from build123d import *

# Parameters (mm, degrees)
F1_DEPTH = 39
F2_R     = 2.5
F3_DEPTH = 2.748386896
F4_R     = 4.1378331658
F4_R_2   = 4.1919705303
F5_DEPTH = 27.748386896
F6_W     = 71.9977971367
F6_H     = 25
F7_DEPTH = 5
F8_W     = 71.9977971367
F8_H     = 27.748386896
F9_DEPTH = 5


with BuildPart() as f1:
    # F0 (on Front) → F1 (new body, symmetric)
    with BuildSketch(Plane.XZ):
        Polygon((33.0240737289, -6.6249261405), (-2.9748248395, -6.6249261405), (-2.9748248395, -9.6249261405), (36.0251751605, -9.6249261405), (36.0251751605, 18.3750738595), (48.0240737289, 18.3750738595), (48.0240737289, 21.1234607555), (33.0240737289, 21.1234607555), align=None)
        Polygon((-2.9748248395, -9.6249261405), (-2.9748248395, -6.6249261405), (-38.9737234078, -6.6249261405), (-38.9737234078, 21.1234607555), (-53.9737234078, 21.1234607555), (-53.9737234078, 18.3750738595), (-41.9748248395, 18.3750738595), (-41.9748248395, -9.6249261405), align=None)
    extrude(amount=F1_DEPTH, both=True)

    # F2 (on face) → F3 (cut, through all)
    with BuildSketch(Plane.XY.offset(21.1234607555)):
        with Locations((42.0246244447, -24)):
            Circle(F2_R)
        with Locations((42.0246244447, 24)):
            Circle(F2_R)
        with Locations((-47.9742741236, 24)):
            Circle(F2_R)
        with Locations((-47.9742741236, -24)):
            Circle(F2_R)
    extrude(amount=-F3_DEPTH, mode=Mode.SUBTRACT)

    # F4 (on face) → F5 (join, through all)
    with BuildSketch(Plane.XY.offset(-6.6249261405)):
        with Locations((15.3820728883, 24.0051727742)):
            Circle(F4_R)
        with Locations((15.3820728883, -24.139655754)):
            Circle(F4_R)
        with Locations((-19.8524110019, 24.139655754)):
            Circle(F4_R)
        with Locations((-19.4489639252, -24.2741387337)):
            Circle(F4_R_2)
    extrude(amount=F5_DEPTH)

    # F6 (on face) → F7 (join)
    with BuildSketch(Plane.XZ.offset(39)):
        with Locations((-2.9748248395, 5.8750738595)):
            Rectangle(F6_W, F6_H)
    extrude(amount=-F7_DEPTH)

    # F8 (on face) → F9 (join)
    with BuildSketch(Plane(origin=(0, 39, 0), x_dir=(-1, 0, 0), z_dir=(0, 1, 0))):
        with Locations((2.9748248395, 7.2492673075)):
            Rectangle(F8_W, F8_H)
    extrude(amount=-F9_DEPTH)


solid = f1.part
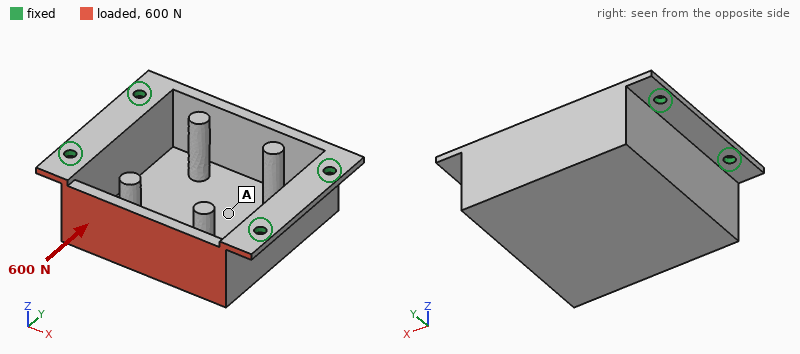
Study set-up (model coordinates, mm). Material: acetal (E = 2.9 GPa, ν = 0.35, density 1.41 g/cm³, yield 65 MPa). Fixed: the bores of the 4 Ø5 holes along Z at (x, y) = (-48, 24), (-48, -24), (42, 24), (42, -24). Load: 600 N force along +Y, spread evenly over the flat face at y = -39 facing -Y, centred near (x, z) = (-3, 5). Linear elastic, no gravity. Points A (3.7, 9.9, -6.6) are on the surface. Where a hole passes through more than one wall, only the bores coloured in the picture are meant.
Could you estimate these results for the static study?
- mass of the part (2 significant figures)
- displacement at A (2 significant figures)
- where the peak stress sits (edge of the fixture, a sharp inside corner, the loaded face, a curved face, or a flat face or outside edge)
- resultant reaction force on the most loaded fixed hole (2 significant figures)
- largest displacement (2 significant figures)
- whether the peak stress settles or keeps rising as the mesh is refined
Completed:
86 g
0.12 mm
edge of the fixture
210 N
0.73 mm
keeps rising
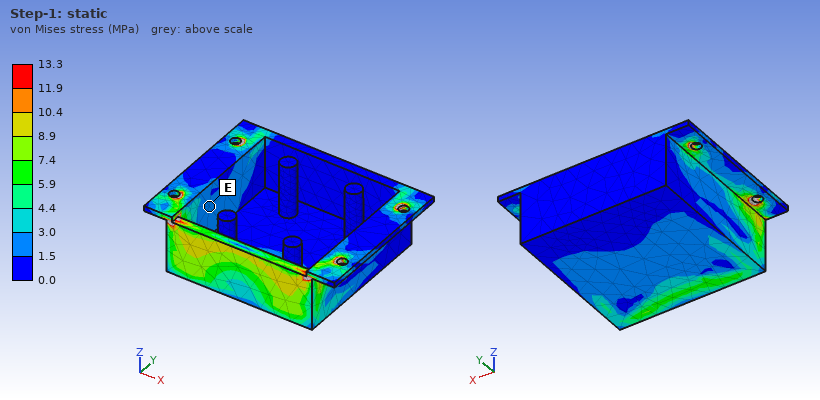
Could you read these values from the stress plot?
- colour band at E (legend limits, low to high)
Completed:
1.5 to 3.0 MPa
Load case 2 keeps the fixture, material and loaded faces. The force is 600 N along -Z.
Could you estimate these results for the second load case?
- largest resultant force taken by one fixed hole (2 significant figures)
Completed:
430 N
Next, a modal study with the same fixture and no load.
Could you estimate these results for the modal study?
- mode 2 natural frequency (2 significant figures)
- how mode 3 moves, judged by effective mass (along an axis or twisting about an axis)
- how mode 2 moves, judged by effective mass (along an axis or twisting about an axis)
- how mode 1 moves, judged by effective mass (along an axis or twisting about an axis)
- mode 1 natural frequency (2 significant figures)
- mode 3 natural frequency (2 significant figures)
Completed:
920 Hz
along X
along Y
along Z
850 Hz
1200 Hz
